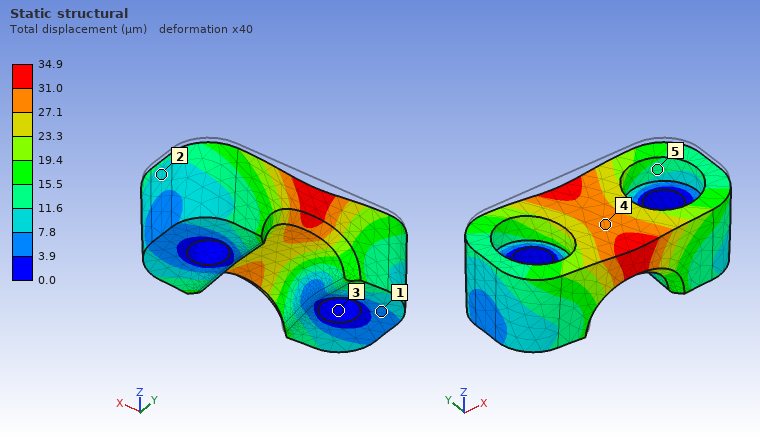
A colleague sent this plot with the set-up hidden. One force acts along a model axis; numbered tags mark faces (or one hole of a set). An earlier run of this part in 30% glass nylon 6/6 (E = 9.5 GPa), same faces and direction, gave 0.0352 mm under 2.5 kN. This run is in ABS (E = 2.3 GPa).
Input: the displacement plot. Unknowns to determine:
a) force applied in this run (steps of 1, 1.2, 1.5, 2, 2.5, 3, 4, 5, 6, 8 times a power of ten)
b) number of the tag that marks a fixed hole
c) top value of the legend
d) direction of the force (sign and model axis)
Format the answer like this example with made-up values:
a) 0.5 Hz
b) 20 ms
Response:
a) 600 N
b) 3
c) 34.9 µm
d) -Z
